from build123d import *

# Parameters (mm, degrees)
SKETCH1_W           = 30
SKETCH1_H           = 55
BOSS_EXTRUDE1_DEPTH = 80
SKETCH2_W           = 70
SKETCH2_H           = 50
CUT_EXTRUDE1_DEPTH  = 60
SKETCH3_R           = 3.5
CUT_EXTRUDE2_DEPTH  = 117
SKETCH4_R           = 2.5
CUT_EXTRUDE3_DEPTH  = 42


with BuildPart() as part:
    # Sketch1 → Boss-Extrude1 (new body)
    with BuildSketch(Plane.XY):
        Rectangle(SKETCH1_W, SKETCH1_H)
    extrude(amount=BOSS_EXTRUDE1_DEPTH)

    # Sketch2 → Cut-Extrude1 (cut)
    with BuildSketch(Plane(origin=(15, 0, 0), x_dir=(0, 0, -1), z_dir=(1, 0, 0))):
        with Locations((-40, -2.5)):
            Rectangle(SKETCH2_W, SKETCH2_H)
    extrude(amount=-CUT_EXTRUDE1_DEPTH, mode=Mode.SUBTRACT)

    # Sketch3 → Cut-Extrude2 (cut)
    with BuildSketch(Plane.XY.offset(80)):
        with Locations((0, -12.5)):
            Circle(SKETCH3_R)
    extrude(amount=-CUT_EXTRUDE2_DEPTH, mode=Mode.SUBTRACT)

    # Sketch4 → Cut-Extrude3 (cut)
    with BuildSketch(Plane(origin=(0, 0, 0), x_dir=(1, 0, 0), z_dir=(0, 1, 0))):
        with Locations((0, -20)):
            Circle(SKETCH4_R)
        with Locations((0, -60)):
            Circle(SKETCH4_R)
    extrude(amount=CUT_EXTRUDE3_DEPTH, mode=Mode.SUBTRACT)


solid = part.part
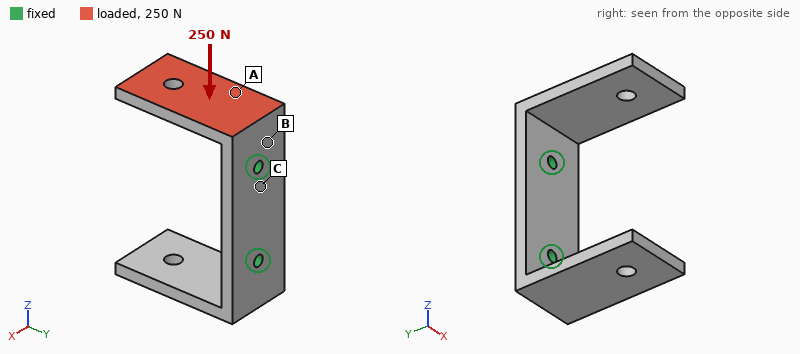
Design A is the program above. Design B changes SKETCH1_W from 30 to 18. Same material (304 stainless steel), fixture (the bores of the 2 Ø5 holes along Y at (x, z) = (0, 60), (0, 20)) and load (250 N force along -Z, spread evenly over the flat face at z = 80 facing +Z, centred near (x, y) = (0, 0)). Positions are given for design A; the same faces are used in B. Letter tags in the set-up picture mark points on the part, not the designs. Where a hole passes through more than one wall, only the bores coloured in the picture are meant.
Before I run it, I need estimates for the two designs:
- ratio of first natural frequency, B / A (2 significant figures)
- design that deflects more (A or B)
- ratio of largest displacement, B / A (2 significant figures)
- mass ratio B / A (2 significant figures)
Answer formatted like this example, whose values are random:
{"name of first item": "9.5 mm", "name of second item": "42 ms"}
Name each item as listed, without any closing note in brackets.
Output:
{"ratio of first natural frequency, B / A": "1.0", "design that deflects more": "B", "ratio of largest displacement, B / A": "1.6", "mass ratio B / A": "0.59"}
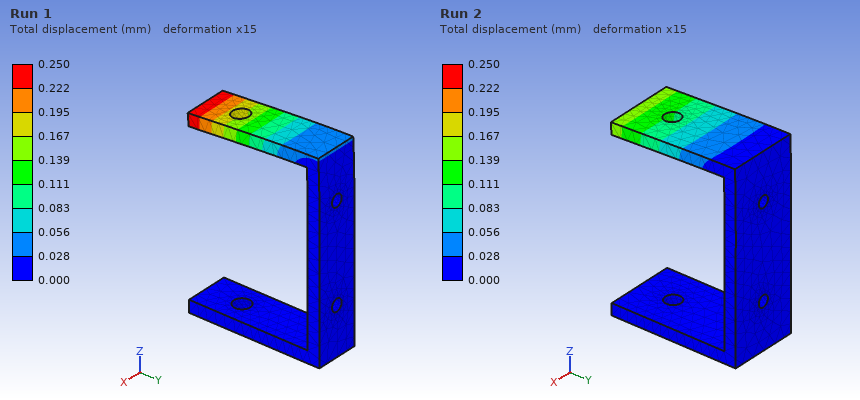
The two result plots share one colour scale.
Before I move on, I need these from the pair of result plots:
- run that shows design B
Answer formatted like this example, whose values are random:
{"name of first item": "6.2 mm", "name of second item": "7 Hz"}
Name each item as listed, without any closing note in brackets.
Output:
{"run that shows design B": "Run 1"}
